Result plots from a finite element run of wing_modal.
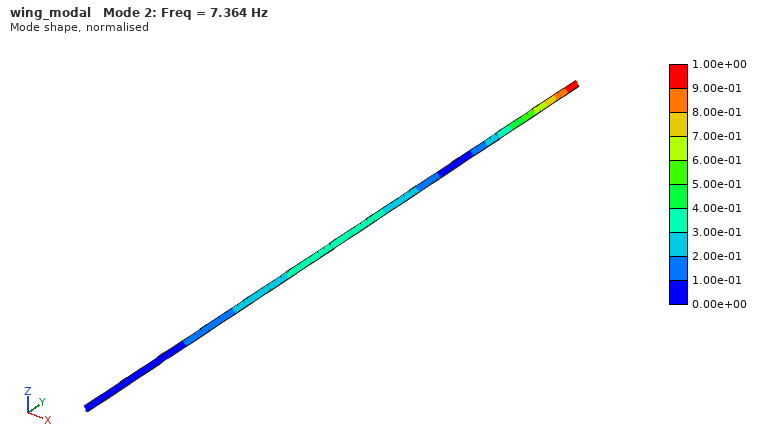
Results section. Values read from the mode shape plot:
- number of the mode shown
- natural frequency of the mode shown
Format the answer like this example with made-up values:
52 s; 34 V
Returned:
2; 7.364 Hz
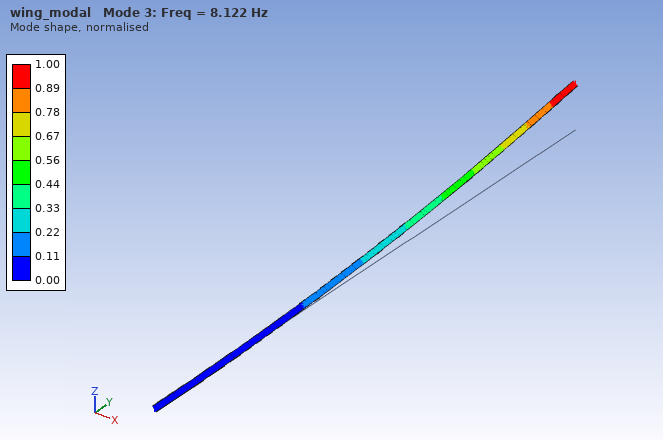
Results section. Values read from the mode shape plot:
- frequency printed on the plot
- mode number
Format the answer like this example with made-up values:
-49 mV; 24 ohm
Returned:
8.122 Hz; 3
